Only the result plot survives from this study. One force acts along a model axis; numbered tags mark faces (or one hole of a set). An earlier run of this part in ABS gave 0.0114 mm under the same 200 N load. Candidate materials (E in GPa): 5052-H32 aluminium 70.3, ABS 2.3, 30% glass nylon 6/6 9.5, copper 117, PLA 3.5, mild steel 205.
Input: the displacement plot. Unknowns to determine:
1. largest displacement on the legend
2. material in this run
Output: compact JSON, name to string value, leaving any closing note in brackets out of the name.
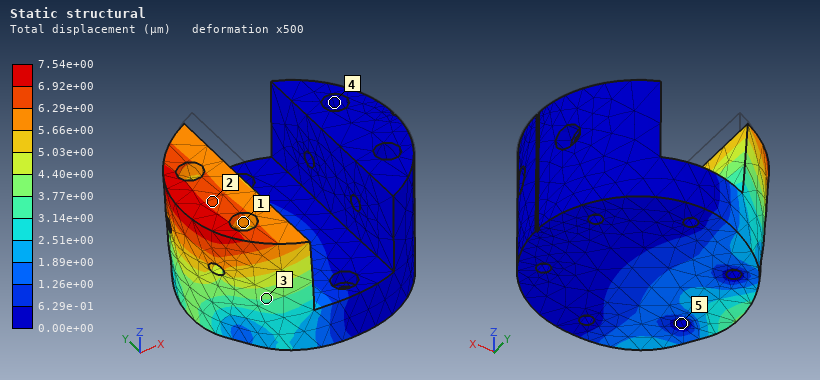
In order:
{"largest displacement on the legend": "7.54e+00 µm", "material in this run": "PLA"}
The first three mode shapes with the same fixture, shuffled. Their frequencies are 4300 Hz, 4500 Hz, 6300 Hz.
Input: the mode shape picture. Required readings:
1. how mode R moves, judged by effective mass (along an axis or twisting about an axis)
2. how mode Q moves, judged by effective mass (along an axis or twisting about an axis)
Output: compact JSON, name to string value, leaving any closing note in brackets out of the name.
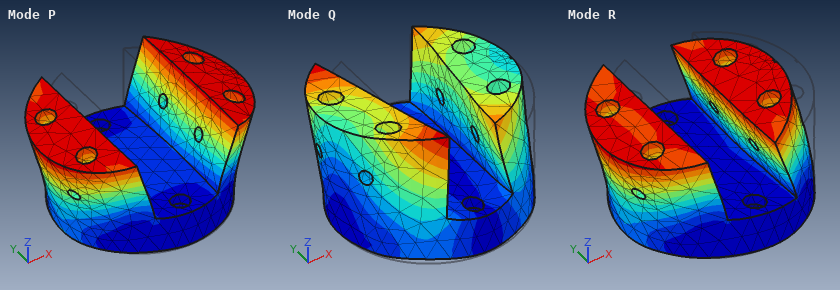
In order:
{"how mode R moves, judged by effective mass": "along X", "how mode Q moves, judged by effective mass": "along Y"}
